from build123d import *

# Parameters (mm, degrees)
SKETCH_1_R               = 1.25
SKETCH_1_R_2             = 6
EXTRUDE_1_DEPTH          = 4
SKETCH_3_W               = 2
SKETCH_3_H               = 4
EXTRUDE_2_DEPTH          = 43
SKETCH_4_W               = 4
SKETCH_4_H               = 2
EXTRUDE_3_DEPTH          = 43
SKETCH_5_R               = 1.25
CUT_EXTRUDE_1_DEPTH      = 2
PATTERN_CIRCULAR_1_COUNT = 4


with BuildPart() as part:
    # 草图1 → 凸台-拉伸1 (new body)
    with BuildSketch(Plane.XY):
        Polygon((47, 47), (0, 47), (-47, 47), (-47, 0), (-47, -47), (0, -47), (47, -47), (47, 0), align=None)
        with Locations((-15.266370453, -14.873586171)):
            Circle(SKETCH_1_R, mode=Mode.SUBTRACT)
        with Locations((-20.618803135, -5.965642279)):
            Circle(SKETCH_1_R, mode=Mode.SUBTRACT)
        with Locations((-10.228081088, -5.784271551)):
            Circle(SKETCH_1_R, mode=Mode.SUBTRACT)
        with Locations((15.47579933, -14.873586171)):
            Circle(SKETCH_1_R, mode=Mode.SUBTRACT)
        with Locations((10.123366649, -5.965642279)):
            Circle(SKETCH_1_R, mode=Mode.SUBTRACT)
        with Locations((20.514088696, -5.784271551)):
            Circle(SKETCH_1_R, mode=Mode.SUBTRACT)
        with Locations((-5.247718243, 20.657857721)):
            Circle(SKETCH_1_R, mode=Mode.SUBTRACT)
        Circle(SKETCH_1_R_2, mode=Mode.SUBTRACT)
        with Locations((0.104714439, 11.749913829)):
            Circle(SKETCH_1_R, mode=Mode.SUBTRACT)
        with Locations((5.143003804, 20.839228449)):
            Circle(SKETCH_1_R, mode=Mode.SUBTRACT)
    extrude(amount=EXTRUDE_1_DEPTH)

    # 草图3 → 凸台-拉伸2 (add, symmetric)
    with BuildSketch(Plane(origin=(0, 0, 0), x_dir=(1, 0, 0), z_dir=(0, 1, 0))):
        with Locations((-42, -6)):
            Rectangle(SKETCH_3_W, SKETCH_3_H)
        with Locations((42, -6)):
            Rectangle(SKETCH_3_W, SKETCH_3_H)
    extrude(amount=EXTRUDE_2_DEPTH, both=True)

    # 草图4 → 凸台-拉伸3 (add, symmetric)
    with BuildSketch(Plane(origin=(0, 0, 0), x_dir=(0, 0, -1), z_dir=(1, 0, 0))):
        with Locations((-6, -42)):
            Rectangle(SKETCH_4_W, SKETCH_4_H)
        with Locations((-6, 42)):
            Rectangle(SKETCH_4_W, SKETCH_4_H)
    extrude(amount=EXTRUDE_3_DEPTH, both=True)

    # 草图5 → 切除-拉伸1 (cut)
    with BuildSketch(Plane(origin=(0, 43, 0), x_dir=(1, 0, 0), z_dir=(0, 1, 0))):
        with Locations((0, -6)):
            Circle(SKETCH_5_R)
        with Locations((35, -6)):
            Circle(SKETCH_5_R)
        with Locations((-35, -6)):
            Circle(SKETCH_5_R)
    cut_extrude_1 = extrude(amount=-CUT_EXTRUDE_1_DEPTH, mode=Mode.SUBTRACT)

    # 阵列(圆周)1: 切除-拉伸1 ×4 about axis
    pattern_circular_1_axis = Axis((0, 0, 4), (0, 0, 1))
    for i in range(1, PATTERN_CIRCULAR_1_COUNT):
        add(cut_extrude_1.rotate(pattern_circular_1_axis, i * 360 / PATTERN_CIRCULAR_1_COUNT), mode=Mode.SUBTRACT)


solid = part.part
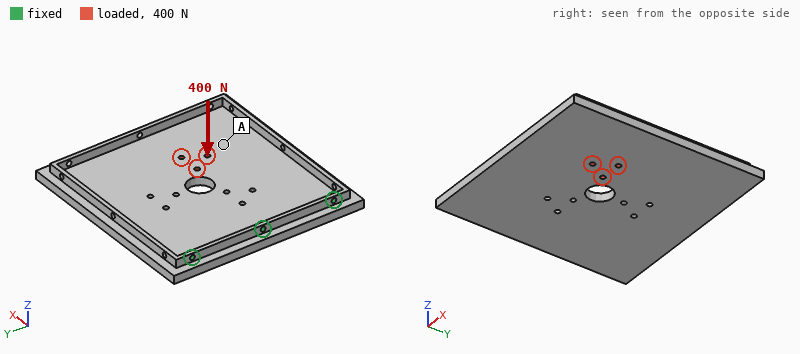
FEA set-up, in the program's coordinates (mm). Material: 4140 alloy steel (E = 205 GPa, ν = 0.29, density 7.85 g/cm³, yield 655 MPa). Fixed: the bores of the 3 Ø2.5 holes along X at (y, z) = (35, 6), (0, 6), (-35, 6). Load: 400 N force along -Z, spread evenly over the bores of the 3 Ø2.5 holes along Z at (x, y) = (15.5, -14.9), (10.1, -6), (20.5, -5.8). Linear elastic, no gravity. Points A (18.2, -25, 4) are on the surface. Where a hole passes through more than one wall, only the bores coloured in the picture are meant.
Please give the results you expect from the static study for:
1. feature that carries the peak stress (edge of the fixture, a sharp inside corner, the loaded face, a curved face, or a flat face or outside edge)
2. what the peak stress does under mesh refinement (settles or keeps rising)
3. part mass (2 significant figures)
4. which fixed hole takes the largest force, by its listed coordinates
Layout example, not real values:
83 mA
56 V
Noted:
edge of the fixture
keeps rising
290 g
(0, 6)
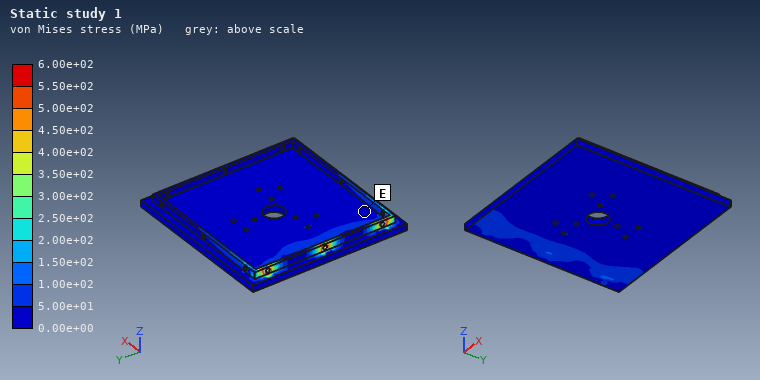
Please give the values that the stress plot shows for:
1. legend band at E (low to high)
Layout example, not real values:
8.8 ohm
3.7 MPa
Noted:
0.00e+00 to 5.00e+01 MPa
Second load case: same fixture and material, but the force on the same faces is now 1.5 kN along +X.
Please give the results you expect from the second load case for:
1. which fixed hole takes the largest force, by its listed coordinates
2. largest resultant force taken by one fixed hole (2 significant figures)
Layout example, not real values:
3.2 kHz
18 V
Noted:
(-35, 6)
690 N
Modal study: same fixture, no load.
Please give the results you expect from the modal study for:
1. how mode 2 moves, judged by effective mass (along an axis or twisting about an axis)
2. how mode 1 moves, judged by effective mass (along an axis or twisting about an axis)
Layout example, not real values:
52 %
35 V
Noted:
twisting about X
along Z
